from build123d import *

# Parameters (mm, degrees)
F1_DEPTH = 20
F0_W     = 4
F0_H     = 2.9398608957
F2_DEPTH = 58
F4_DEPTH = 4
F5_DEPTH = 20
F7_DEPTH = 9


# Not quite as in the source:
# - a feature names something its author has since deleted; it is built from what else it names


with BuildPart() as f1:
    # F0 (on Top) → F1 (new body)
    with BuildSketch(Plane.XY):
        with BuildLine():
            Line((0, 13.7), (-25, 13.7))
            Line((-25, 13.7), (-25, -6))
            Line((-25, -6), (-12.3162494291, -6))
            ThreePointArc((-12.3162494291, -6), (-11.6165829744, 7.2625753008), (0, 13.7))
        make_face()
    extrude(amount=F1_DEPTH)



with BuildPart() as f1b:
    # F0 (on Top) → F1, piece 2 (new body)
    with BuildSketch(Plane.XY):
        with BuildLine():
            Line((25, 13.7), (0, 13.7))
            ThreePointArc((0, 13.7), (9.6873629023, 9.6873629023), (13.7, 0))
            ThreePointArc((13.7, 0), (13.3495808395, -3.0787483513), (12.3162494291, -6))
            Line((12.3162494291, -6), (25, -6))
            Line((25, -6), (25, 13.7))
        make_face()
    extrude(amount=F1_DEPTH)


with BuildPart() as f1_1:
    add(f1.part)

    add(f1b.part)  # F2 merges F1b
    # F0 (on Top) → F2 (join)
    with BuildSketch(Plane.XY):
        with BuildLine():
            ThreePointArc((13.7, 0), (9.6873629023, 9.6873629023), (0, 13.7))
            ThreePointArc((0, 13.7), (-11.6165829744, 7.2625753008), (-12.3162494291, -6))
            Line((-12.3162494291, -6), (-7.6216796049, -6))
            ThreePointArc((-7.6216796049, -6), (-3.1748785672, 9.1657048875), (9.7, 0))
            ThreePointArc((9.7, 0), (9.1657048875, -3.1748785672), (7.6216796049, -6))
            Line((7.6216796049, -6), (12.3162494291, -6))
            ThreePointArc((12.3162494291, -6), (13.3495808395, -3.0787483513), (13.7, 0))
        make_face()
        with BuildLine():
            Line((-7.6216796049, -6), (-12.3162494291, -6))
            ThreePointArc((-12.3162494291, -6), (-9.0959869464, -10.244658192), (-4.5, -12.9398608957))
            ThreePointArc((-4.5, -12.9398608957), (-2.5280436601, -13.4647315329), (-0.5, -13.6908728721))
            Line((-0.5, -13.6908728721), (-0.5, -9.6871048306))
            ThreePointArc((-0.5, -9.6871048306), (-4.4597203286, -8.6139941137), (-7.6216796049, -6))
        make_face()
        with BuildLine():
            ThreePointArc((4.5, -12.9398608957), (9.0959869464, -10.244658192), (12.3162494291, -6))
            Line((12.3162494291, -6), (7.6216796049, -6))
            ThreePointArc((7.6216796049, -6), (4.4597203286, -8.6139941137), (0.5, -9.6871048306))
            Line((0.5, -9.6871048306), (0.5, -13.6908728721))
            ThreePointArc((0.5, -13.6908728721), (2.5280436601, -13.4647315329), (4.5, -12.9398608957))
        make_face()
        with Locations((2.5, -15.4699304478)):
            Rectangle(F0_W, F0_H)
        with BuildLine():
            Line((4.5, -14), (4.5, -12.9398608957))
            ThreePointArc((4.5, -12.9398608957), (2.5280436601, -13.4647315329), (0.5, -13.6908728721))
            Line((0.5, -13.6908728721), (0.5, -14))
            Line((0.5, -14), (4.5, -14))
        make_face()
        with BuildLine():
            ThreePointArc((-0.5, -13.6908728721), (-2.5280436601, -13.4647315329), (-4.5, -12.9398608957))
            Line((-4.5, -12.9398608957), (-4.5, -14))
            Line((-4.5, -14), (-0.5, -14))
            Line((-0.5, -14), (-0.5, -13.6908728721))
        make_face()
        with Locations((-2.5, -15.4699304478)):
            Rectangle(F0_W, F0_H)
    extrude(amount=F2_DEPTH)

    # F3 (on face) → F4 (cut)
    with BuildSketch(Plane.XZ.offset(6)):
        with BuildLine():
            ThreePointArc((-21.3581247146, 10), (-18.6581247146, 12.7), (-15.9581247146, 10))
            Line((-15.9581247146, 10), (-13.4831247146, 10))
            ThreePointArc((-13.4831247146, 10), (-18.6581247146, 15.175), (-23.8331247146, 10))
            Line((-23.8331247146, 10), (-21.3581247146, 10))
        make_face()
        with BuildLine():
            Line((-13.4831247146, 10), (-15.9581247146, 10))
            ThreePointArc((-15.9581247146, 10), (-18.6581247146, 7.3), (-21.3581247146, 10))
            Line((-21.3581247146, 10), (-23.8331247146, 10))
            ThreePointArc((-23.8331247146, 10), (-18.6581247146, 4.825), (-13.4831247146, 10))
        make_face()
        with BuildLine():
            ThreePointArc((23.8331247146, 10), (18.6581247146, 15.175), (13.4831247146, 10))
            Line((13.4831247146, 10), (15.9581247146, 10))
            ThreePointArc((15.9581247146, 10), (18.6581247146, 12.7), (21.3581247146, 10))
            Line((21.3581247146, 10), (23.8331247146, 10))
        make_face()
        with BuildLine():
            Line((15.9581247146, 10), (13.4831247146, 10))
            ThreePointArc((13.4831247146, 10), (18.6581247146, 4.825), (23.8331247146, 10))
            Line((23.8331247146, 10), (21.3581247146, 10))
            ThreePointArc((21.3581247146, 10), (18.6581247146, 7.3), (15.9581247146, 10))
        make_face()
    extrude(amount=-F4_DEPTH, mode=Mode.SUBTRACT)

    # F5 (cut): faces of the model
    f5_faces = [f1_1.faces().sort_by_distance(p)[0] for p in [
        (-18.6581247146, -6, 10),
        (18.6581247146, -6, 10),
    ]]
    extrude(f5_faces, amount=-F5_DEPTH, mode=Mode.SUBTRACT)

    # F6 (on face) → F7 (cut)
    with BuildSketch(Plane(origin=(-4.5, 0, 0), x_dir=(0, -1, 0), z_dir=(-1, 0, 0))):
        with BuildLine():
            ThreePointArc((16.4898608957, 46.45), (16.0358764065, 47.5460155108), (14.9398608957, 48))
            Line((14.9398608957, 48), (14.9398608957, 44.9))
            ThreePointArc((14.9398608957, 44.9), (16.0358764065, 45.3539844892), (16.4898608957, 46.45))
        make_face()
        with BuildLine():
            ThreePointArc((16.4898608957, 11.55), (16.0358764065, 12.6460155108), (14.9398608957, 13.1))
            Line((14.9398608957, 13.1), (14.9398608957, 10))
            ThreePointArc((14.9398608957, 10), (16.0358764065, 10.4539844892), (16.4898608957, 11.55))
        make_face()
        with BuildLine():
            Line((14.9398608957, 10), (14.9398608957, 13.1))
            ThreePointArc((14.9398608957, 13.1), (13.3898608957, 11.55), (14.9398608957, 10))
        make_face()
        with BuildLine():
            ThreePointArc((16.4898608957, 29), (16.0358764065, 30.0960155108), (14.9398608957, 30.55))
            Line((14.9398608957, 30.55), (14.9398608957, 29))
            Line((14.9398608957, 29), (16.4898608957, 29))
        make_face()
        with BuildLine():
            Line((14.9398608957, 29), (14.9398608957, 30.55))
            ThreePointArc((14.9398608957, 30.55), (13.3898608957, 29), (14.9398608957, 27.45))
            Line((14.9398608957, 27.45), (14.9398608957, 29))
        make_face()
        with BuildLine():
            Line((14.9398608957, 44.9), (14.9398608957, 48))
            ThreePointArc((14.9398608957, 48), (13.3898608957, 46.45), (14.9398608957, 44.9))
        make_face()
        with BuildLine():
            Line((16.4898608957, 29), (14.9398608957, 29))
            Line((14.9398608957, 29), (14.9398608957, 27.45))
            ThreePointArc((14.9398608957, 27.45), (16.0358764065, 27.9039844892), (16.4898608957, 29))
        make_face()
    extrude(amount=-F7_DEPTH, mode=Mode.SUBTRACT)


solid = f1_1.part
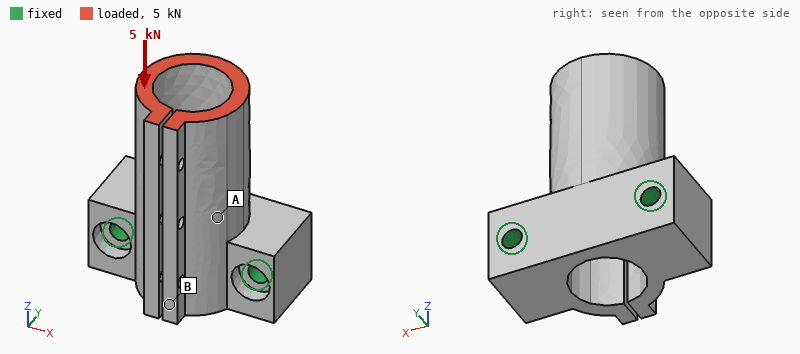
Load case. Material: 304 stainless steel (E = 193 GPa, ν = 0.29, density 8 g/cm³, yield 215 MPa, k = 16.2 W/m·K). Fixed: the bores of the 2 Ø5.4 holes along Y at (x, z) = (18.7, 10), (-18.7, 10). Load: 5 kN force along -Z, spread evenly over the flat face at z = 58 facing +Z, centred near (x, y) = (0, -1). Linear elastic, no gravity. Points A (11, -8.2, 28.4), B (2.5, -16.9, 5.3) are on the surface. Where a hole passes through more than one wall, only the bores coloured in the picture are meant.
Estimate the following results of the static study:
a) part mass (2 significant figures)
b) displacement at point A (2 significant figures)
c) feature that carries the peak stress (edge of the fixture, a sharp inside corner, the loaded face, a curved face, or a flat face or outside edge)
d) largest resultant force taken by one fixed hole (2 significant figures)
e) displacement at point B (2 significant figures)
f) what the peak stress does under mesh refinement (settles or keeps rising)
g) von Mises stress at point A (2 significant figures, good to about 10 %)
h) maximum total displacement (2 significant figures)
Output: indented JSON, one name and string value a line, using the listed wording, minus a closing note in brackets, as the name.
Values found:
{
  "part mass": "220 g",
  "displacement at point A": "8.1 µm",
  "feature that carries the peak stress": "edge of the fixture",
  "largest resultant force taken by one fixed hole": "2.5 kN",
  "displacement at point B": "8.1 µm",
  "what the peak stress does under mesh refinement": "keeps rising",
  "von Mises stress at point A": "22 MPa",
  "maximum total displacement": "19 µm"
}
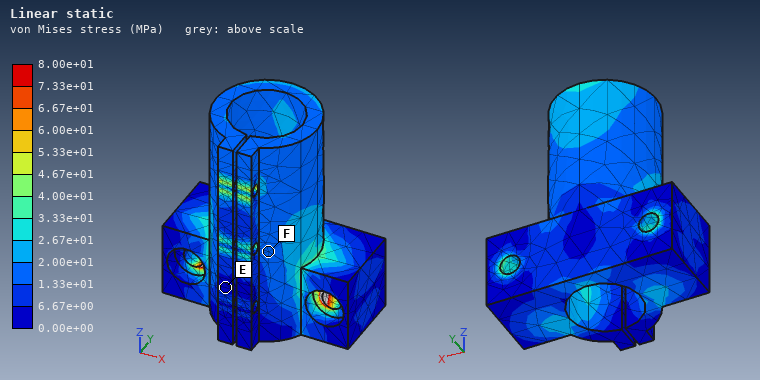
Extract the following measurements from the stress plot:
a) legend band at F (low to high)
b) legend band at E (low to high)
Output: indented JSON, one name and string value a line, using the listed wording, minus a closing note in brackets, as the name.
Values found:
{
  "legend band at F": "1.33e+01 to 2.00e+01 MPa",
  "legend band at E": "0.00e+00 to 6.67e+00 MPa"
}
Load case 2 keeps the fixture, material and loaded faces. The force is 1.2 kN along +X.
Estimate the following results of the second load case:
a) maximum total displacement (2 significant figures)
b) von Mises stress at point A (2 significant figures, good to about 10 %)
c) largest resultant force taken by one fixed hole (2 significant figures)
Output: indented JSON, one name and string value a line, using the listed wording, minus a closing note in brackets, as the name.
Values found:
{
  "maximum total displacement": "63 µm",
  "von Mises stress at point A": "25 MPa",
  "largest resultant force taken by one fixed hole": "1.4 kN"
}
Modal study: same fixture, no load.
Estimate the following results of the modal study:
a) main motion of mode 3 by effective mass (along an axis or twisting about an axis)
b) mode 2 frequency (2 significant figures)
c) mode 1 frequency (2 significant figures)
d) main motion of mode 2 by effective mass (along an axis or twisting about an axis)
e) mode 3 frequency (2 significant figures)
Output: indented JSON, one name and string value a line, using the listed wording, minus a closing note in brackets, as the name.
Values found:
{
  "main motion of mode 3 by effective mass": "along Y",
  "mode 2 frequency": "4300 Hz",
  "mode 1 frequency": "4000 Hz",
  "main motion of mode 2 by effective mass": "along X",
  "mode 3 frequency": "5700 Hz"
}
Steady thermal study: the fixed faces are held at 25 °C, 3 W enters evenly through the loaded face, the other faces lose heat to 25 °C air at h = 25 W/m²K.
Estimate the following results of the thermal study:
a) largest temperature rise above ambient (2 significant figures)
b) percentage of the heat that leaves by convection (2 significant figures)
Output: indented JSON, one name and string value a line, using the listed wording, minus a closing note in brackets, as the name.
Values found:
{
  "largest temperature rise above ambient": "18 K",
  "percentage of the heat that leaves by convection": "56 %"
}
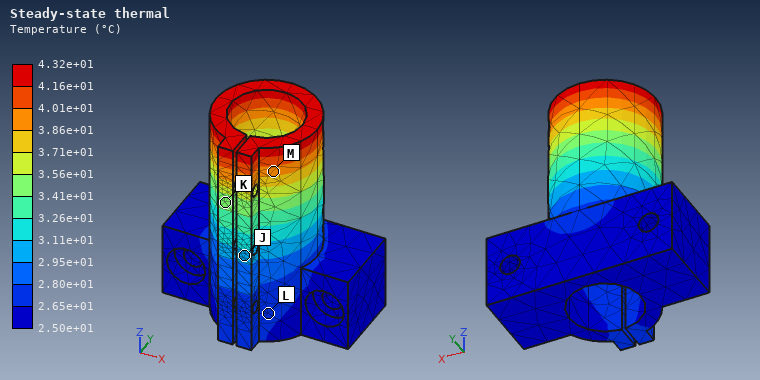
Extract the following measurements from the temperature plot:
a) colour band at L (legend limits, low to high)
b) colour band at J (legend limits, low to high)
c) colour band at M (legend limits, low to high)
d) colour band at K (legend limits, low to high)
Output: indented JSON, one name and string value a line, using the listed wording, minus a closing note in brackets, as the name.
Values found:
{
  "colour band at L": "2.65e+01 to 2.80e+01 °C",
  "colour band at J": "2.95e+01 to 3.11e+01 °C",
  "colour band at M": "3.86e+01 to 4.01e+01 °C",
  "colour band at K": "3.41e+01 to 3.56e+01 °C"
}
